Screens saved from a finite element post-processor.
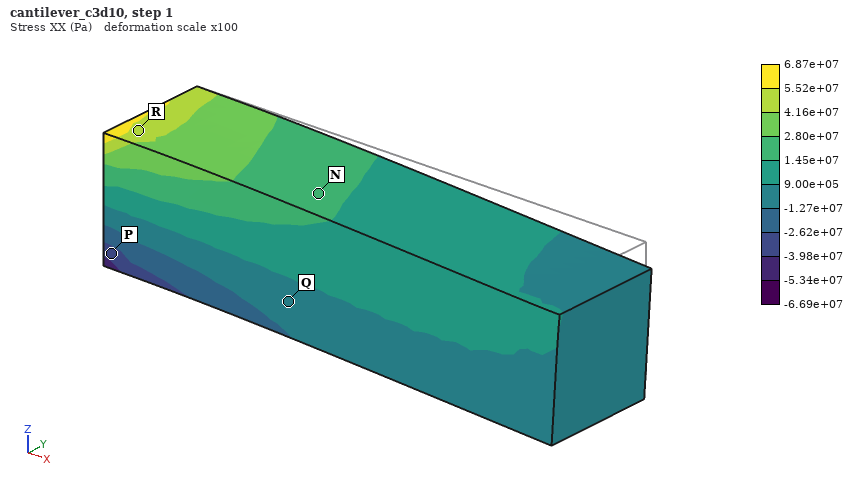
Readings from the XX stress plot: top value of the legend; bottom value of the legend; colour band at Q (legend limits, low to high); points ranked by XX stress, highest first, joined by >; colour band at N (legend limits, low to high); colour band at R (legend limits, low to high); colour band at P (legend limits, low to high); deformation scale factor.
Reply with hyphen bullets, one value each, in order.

- 6.87e+07 Pa
- -6.69e+07 Pa
- -1.27e+07 to 9.00e+05 Pa
- R > N > Q > P
- 1.45e+07 to 2.80e+07 Pa
- 4.16e+07 to 5.52e+07 Pa
- -3.98e+07 to -2.62e+07 Pa
- 100
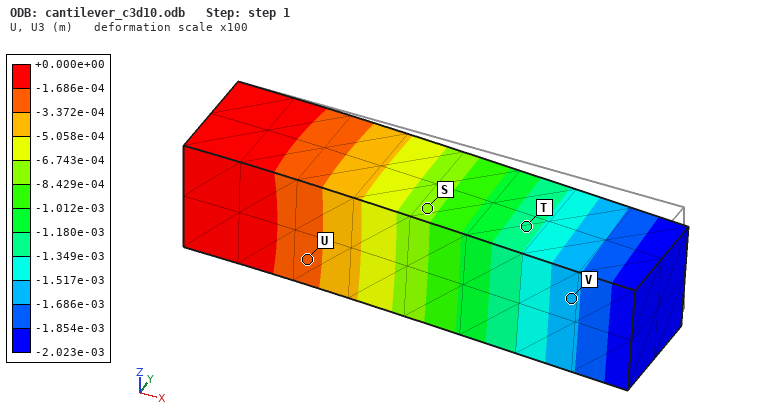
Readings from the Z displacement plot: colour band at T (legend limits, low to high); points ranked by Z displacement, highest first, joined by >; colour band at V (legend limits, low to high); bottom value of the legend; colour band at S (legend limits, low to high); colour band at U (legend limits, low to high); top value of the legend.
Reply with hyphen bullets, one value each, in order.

- -1.349e-03 to -1.180e-03 m
- U > S > T > V
- -1.686e-03 to -1.517e-03 m
- -2.023e-03 m
- -8.429e-04 to -6.743e-04 m
- -3.372e-04 to -1.686e-04 m
- +0.000e+00 m
